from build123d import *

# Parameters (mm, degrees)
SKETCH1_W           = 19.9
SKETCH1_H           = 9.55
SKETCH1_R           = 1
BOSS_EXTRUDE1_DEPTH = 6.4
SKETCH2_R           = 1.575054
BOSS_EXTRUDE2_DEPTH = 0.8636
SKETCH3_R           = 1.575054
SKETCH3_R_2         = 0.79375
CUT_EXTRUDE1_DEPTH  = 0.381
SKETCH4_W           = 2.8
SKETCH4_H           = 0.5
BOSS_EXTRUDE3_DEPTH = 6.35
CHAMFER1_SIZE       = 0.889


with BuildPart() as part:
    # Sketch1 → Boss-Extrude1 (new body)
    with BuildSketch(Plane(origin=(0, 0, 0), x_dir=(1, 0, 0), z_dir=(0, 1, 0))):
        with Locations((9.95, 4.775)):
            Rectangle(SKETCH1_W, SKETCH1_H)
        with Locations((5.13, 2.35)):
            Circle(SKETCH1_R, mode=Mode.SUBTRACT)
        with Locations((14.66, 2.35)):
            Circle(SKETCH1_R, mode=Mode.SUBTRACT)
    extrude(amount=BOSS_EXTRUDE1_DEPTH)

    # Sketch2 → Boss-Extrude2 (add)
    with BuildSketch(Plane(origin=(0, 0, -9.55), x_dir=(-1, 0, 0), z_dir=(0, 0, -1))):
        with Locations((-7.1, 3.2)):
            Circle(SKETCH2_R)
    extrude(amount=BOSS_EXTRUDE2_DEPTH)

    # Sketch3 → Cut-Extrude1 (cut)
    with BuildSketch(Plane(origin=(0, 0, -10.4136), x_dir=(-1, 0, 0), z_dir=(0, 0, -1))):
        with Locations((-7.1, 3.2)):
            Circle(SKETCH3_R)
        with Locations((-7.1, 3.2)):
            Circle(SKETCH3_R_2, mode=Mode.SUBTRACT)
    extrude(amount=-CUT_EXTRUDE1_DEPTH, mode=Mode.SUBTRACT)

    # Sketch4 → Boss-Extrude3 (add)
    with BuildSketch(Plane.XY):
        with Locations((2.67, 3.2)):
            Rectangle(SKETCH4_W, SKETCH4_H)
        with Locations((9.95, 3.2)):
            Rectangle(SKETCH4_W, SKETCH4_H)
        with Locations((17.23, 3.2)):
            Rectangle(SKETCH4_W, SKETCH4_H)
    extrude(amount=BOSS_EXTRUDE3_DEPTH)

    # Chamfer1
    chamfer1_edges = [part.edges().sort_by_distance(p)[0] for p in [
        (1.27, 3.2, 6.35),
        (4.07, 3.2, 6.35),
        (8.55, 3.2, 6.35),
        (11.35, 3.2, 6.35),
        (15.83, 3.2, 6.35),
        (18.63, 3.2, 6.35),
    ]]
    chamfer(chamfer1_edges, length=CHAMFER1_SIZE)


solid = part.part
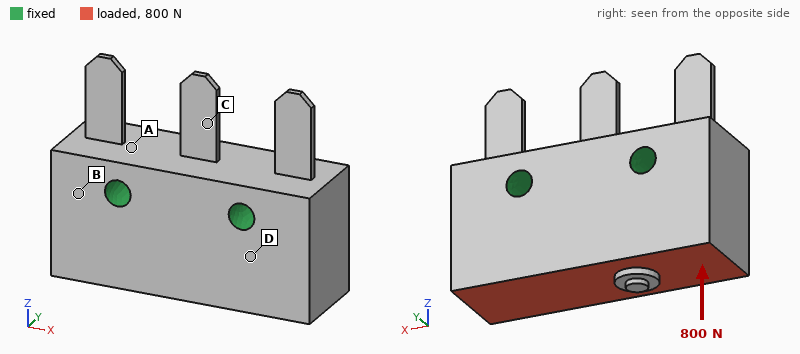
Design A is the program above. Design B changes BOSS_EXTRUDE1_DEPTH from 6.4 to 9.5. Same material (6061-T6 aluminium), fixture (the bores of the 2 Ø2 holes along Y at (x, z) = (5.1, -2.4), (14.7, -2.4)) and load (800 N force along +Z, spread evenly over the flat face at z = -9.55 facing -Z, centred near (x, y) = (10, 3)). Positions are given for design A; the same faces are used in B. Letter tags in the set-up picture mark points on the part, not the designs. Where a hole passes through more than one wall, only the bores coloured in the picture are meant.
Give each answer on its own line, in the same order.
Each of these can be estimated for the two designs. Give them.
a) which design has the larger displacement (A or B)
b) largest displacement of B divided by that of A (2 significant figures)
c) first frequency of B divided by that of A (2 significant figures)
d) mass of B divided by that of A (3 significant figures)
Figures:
A
0.65
1.00
1.47
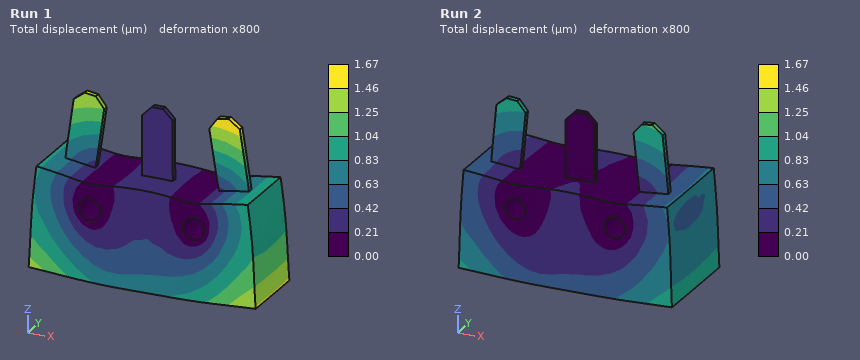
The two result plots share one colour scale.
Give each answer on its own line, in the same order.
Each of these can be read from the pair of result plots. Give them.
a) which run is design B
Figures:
Run 2
